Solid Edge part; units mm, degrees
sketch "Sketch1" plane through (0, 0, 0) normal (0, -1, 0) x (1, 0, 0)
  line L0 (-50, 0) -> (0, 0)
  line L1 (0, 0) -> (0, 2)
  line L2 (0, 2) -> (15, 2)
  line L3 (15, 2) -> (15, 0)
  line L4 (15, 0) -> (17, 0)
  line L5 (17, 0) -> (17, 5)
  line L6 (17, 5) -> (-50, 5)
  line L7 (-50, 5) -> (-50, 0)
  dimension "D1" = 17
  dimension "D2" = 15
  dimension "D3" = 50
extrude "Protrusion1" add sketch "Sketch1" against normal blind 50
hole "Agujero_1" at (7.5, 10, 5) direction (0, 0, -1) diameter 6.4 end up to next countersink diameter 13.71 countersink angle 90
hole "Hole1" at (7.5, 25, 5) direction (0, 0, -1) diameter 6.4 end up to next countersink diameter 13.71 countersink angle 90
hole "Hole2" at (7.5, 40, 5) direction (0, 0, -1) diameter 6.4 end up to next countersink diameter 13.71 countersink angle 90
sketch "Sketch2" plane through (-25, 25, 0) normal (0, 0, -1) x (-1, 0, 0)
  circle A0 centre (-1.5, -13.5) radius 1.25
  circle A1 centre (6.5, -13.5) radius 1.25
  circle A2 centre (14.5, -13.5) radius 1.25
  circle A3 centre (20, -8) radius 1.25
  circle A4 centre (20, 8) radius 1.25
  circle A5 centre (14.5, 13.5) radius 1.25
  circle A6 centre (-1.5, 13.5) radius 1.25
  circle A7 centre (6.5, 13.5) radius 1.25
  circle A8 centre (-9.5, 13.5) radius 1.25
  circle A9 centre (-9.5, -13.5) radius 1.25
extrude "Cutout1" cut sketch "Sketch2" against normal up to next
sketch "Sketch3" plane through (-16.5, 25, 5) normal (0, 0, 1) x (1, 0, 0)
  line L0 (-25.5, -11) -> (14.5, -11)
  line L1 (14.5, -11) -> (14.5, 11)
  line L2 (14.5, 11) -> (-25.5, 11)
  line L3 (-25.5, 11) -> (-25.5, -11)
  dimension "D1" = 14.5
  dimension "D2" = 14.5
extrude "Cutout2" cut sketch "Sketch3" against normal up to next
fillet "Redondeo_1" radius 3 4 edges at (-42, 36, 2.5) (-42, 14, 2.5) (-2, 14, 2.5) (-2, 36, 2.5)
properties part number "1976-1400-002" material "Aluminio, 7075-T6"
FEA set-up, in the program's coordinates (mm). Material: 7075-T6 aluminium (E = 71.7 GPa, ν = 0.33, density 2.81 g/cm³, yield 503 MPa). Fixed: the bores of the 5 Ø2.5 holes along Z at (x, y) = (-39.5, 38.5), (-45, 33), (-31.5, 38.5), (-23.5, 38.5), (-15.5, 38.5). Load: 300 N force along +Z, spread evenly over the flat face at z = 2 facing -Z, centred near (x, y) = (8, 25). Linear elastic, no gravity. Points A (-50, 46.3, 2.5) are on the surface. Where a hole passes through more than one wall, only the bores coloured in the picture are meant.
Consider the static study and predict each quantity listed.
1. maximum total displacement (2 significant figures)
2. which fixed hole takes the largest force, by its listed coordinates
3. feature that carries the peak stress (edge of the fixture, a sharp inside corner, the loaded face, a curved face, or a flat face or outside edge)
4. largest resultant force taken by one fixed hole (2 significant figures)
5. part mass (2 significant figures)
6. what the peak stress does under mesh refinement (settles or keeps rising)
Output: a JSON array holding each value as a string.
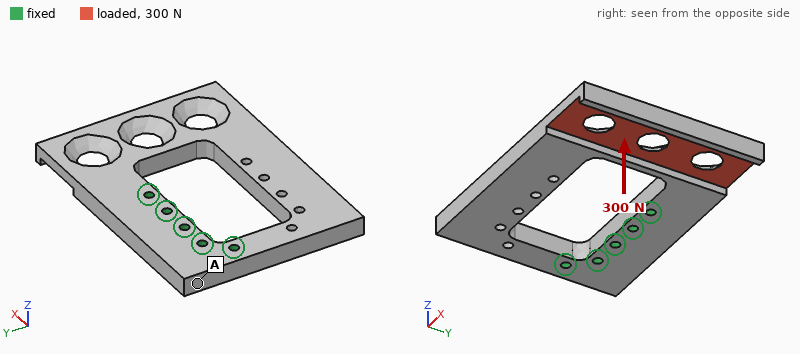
["0.67 mm", "(-15.5, 38.5)", "edge of the fixture", "510 N", "28 g", "keeps rising"]
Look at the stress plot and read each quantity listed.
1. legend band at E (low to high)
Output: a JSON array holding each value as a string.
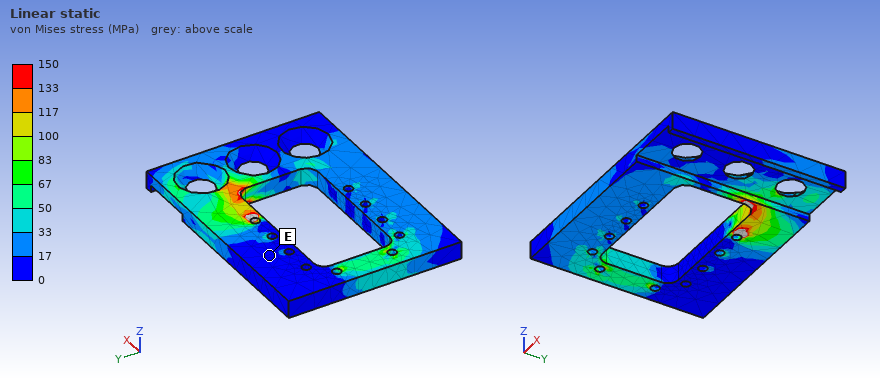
["0 to 17 MPa"]
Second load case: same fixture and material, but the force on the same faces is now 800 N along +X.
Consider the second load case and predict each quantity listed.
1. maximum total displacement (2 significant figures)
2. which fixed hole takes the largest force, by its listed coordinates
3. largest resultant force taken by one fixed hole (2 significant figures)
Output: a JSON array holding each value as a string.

["78 µm", "(-15.5, 38.5)", "710 N"]
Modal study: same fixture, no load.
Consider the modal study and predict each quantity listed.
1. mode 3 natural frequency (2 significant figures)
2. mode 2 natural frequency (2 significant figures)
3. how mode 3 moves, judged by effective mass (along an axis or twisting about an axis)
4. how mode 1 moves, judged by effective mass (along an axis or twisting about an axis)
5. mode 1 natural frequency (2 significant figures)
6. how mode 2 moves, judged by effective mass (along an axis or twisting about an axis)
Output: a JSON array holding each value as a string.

["4000 Hz", "2600 Hz", "along X", "along Z", "1200 Hz", "twisting about Y"]
